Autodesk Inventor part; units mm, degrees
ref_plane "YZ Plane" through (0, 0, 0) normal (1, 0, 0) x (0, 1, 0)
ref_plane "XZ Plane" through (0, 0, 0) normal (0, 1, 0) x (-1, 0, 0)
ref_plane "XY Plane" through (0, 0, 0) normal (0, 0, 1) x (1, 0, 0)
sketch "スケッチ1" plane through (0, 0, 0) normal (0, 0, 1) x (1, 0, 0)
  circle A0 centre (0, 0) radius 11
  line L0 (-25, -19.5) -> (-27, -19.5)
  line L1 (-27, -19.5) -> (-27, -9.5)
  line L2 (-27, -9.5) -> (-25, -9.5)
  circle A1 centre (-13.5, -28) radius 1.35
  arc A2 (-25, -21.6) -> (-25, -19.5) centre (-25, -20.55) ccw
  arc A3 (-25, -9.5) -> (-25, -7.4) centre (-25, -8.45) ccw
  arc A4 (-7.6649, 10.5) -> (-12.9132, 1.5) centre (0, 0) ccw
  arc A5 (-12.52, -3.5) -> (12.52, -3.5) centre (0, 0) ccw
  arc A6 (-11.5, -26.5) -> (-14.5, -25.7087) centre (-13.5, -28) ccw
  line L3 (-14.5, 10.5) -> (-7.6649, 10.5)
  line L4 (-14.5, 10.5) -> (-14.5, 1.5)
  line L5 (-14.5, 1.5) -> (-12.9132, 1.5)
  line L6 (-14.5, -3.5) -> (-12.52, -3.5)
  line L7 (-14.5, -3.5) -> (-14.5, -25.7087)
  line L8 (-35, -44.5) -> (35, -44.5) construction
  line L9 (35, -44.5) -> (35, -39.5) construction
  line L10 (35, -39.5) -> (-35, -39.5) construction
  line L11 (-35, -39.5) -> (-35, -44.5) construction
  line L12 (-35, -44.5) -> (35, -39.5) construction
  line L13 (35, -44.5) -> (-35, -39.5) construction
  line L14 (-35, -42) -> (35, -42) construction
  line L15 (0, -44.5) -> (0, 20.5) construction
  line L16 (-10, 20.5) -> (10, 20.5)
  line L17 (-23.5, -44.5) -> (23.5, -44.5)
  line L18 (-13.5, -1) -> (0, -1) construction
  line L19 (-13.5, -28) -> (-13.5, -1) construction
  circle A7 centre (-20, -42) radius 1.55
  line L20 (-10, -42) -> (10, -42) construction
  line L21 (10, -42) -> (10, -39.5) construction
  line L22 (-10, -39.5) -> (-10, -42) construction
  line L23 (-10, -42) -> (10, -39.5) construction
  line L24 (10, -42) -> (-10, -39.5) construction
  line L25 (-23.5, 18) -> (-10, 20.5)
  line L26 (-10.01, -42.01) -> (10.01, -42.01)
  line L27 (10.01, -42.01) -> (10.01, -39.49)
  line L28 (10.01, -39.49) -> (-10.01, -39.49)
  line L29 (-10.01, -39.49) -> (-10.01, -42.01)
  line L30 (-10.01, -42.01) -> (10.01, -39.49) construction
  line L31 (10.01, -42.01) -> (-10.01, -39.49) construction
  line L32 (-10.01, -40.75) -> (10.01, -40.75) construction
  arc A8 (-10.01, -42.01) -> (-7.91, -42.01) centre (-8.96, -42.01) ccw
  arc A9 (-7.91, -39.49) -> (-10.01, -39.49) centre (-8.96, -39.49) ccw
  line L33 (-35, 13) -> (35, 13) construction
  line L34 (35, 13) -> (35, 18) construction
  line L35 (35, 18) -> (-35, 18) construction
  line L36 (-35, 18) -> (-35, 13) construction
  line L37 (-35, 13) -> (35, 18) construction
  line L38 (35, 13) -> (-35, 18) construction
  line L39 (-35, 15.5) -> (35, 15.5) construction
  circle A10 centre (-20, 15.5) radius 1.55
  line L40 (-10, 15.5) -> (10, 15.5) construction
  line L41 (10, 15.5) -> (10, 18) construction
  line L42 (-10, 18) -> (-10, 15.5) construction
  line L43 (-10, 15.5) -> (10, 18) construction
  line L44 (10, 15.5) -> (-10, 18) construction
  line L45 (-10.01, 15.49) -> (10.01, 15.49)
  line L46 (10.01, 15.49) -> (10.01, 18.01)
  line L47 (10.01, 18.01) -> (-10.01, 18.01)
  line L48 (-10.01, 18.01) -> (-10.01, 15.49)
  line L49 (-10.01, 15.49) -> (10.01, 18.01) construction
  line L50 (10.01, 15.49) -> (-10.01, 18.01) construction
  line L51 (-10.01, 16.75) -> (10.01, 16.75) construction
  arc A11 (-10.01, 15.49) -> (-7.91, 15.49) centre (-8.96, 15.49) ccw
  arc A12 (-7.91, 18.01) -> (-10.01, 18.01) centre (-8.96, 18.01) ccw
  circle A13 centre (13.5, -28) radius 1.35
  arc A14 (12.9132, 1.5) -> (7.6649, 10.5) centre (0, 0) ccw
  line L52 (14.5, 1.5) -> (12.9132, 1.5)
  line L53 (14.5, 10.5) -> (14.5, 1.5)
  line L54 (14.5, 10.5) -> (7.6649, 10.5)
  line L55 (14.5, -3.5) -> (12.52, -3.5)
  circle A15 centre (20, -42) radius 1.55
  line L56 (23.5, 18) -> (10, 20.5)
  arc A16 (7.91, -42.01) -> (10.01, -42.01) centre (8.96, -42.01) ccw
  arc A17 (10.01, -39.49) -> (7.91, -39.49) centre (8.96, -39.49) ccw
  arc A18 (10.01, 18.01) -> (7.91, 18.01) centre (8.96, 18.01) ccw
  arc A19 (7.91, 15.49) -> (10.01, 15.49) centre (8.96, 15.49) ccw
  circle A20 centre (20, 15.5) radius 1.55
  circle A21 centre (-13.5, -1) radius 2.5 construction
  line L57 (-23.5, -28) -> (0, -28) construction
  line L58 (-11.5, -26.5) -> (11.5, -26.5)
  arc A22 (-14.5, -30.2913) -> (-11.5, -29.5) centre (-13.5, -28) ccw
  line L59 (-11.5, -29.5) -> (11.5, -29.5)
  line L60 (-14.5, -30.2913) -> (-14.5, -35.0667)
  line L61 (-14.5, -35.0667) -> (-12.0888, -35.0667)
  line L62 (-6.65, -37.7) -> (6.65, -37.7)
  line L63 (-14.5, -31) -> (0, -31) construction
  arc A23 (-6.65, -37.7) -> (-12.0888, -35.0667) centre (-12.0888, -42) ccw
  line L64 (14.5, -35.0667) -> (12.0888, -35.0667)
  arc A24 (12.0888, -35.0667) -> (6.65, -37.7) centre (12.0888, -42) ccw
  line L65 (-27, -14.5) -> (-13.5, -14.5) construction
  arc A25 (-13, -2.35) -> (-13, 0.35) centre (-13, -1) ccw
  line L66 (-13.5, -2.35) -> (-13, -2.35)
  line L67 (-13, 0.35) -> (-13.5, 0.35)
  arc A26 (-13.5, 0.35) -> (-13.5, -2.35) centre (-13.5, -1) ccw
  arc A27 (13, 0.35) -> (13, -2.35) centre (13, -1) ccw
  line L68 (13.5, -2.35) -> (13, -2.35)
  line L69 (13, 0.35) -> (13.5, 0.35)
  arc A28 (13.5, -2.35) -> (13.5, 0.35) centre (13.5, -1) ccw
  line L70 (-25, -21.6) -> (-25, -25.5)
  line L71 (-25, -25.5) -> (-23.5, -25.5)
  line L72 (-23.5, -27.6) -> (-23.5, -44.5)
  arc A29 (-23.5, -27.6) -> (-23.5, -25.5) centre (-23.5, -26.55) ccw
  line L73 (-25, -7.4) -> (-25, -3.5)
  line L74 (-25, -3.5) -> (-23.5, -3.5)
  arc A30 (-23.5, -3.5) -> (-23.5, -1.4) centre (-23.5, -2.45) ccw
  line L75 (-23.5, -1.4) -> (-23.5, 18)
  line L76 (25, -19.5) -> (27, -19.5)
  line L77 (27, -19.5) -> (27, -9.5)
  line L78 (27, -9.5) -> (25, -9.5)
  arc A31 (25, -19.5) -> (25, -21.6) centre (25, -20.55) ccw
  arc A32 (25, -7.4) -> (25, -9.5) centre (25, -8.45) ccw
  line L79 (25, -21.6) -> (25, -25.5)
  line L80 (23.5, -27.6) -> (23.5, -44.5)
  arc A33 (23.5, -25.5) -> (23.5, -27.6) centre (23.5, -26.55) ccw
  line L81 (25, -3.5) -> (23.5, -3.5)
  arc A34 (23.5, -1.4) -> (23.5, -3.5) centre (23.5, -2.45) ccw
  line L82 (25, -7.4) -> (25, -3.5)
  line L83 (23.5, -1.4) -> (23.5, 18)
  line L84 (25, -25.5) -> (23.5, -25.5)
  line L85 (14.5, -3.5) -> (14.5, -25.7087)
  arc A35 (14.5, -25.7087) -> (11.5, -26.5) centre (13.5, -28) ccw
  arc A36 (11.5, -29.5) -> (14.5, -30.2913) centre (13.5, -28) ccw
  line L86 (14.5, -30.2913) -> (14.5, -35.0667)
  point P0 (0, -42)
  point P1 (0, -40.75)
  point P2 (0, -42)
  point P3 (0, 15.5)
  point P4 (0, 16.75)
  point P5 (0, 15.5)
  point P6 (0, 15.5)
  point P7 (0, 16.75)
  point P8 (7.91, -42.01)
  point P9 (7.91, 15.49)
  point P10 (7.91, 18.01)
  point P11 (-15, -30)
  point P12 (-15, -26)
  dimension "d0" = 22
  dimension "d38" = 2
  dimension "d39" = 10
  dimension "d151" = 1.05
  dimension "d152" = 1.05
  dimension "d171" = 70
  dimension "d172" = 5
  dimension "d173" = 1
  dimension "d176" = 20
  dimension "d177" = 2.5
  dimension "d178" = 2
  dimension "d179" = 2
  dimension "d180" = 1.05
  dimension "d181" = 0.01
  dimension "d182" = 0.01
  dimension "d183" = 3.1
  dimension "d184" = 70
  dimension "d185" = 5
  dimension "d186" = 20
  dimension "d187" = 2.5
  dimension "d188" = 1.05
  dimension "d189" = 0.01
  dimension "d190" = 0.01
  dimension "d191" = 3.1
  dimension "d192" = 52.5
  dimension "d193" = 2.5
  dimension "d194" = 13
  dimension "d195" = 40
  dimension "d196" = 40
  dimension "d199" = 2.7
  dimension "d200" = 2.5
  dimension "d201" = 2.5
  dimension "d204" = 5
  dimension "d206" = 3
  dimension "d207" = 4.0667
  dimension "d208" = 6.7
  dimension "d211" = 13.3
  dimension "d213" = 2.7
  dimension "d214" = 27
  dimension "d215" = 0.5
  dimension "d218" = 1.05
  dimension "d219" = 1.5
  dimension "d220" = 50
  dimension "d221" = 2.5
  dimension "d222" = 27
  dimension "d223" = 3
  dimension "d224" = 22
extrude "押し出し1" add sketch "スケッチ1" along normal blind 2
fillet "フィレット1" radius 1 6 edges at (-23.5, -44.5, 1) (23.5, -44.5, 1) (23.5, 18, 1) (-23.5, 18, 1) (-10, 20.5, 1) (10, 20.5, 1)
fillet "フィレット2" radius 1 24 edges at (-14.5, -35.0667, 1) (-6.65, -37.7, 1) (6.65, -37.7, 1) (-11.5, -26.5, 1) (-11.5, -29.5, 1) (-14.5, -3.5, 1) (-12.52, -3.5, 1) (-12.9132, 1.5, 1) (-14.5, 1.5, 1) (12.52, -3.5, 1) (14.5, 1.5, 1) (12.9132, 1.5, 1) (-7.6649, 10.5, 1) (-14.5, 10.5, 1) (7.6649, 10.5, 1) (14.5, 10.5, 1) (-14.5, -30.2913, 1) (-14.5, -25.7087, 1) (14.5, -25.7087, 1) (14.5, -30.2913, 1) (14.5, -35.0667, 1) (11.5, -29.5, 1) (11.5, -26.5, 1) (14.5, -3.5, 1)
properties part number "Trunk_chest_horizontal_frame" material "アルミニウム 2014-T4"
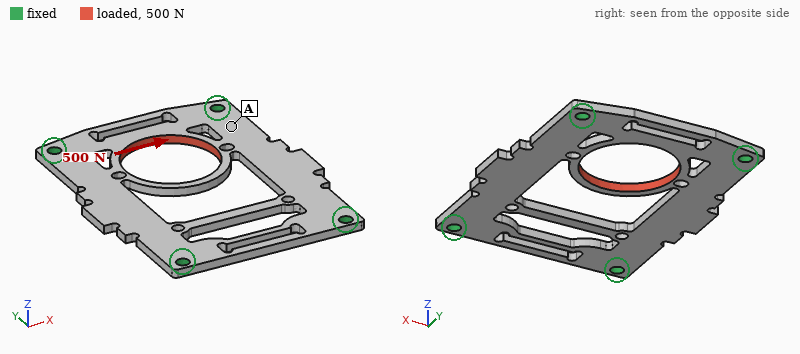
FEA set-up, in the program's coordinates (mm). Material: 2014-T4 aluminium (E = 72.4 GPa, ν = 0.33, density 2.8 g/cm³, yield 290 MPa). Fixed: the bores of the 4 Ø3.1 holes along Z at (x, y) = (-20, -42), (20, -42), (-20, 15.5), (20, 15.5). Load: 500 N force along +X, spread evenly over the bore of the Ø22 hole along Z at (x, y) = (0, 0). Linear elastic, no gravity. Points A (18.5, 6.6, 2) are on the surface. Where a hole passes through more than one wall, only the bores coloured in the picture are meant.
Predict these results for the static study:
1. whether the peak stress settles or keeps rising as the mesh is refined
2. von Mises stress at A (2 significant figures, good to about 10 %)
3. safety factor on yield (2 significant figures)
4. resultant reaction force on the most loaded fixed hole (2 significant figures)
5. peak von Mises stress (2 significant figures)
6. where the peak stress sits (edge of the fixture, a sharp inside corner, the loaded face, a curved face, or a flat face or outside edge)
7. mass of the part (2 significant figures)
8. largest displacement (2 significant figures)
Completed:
settles
15 MPa
1.1
240 N
250 MPa
a curved face
10 g
64 µm
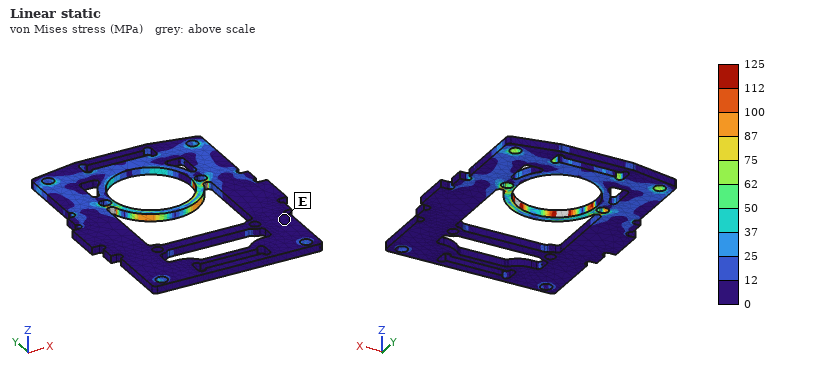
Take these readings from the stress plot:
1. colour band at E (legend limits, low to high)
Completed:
0 to 12 MPa
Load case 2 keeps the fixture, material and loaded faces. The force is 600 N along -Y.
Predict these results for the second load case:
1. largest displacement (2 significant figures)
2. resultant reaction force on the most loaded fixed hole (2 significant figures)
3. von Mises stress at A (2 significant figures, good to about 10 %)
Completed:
19 µm
250 N
13 MPa
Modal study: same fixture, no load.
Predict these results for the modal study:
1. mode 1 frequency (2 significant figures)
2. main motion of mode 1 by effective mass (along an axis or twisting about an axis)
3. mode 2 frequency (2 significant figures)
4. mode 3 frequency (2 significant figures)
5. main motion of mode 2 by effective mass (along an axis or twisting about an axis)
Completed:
2800 Hz
along Z
3300 Hz
4600 Hz
twisting about Y
